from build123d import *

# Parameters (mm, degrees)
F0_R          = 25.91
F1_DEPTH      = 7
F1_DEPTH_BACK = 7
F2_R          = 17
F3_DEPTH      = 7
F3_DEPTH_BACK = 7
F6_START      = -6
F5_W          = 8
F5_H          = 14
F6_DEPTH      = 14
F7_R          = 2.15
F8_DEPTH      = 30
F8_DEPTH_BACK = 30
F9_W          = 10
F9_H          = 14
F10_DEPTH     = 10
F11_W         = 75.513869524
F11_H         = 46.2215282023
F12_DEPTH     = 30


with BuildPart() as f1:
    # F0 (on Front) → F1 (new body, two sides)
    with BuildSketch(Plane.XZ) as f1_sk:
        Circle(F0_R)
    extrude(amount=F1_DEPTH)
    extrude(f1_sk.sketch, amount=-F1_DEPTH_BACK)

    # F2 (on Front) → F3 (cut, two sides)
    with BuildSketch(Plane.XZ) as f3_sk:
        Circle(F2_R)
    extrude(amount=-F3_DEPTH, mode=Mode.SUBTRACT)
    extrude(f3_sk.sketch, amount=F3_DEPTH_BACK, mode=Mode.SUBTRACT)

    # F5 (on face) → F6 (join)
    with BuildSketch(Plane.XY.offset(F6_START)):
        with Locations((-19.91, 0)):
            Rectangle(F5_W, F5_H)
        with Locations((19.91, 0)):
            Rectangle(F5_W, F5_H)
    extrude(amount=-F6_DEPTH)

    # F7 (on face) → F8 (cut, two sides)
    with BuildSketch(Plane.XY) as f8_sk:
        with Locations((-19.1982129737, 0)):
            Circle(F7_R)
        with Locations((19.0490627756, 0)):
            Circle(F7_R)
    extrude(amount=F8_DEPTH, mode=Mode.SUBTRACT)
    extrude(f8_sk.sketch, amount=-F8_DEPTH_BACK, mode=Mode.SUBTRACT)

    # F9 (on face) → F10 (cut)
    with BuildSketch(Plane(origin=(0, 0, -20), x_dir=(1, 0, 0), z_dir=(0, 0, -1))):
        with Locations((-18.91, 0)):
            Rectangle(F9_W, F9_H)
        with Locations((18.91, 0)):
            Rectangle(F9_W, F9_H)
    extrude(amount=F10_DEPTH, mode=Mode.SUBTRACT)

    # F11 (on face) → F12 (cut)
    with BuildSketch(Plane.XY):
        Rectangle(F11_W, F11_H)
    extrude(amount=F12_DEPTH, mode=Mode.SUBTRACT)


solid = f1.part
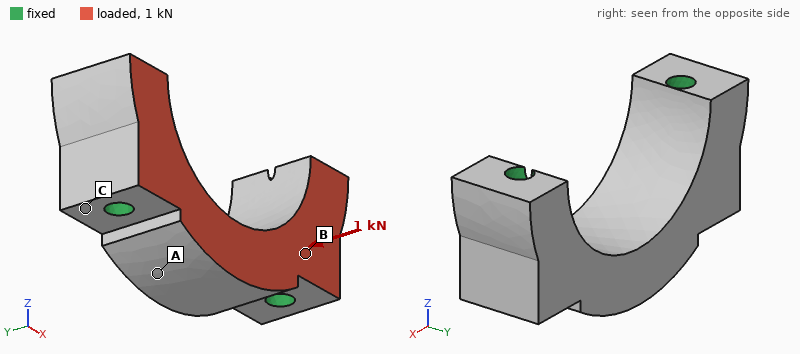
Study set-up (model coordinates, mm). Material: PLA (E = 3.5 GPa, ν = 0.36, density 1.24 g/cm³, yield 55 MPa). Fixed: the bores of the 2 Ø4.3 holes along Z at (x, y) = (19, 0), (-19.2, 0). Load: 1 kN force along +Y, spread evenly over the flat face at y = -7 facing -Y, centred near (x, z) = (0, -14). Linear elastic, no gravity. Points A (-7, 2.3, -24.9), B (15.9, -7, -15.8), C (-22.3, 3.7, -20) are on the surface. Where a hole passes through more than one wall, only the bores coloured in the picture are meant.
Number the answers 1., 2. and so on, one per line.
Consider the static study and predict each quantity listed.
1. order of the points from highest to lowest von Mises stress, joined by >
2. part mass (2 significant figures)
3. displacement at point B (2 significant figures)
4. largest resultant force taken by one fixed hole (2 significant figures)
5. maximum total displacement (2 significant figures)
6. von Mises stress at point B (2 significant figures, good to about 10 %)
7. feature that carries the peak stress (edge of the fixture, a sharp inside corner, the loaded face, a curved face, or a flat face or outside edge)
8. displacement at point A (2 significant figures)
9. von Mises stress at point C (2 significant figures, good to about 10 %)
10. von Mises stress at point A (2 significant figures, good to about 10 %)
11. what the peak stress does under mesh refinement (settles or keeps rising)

1. B > A > C
2. 11 g
3. 15 µm
4. 500 N
5. 62 µm
6. 4.8 MPa
7. edge of the fixture
8. 48 µm
9. 1.4 MPa
10. 2.8 MPa
11. keeps rising
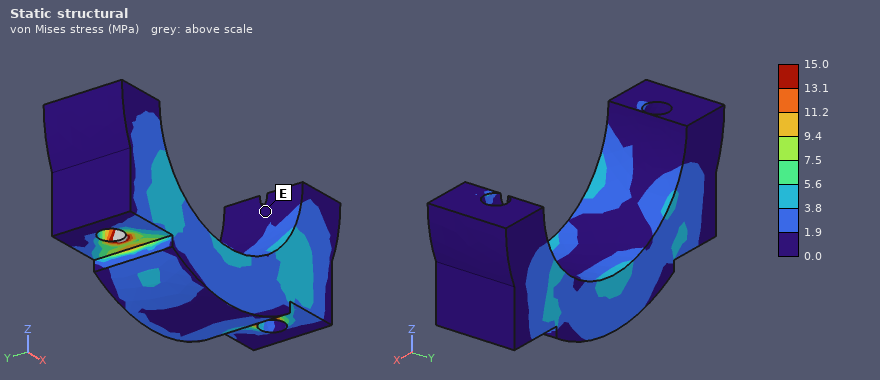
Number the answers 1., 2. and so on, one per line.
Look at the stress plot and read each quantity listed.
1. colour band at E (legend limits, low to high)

1. 0.0 to 1.9 MPa
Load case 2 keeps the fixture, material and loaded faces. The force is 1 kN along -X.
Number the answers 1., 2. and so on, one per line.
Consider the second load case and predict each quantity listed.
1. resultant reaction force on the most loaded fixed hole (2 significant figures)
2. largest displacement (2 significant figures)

1. 510 N
2. 22 µm
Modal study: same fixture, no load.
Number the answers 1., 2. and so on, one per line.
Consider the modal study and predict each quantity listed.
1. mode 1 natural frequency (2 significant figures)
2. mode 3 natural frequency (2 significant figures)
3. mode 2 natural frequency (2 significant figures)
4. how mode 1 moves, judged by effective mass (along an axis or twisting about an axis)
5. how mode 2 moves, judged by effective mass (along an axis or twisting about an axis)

1. 7400 Hz
2. 15 kHz
3. 11 kHz
4. along Y
5. along Z
